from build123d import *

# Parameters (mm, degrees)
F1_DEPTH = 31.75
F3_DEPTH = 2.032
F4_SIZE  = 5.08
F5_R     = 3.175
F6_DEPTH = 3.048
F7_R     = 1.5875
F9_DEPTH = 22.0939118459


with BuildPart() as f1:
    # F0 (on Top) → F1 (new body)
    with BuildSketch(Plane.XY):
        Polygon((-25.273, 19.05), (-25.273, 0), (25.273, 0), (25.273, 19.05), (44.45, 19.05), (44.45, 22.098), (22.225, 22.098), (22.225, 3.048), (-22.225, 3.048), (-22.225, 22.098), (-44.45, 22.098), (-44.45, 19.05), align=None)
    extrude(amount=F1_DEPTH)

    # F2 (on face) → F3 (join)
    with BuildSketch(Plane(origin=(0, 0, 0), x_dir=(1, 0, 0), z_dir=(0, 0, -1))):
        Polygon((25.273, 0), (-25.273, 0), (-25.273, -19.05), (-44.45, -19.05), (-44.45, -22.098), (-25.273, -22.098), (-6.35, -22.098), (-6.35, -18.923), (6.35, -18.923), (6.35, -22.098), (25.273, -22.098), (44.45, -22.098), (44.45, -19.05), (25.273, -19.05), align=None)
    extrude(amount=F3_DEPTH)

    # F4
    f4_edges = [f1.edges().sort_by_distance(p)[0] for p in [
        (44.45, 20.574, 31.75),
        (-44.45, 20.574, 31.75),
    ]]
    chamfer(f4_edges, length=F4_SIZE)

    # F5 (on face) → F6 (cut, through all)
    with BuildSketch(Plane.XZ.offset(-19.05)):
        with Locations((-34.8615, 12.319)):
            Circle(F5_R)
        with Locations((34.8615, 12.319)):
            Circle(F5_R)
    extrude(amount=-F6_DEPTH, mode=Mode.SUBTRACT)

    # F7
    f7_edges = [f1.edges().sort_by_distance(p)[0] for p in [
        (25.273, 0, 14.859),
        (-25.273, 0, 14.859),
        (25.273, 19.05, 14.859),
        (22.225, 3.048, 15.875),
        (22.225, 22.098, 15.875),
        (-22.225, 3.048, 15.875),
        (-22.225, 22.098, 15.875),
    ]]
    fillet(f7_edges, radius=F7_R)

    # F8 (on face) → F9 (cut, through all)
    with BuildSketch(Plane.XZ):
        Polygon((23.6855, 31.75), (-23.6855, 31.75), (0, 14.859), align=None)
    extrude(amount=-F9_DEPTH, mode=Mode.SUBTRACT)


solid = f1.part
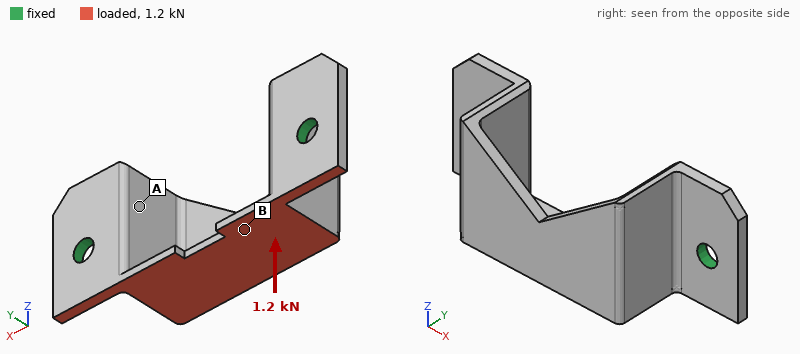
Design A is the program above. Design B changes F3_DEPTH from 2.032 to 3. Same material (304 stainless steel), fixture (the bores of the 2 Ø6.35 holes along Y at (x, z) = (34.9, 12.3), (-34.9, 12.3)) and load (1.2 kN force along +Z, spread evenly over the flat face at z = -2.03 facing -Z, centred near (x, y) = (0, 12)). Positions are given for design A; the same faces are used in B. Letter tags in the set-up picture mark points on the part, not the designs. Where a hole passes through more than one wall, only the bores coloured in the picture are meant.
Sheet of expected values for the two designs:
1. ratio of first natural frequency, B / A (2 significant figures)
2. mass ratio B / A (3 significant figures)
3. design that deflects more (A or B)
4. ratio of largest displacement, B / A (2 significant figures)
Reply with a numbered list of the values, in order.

1. 0.95
2. 1.09
3. A
4. 0.82
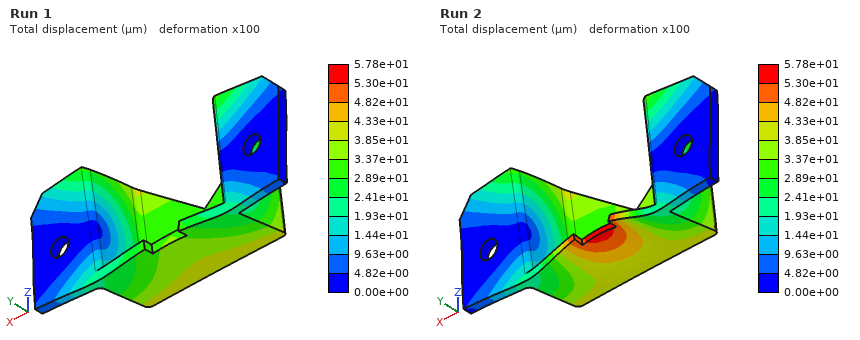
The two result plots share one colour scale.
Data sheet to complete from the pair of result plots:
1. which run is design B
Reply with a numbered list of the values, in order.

1. Run 1
